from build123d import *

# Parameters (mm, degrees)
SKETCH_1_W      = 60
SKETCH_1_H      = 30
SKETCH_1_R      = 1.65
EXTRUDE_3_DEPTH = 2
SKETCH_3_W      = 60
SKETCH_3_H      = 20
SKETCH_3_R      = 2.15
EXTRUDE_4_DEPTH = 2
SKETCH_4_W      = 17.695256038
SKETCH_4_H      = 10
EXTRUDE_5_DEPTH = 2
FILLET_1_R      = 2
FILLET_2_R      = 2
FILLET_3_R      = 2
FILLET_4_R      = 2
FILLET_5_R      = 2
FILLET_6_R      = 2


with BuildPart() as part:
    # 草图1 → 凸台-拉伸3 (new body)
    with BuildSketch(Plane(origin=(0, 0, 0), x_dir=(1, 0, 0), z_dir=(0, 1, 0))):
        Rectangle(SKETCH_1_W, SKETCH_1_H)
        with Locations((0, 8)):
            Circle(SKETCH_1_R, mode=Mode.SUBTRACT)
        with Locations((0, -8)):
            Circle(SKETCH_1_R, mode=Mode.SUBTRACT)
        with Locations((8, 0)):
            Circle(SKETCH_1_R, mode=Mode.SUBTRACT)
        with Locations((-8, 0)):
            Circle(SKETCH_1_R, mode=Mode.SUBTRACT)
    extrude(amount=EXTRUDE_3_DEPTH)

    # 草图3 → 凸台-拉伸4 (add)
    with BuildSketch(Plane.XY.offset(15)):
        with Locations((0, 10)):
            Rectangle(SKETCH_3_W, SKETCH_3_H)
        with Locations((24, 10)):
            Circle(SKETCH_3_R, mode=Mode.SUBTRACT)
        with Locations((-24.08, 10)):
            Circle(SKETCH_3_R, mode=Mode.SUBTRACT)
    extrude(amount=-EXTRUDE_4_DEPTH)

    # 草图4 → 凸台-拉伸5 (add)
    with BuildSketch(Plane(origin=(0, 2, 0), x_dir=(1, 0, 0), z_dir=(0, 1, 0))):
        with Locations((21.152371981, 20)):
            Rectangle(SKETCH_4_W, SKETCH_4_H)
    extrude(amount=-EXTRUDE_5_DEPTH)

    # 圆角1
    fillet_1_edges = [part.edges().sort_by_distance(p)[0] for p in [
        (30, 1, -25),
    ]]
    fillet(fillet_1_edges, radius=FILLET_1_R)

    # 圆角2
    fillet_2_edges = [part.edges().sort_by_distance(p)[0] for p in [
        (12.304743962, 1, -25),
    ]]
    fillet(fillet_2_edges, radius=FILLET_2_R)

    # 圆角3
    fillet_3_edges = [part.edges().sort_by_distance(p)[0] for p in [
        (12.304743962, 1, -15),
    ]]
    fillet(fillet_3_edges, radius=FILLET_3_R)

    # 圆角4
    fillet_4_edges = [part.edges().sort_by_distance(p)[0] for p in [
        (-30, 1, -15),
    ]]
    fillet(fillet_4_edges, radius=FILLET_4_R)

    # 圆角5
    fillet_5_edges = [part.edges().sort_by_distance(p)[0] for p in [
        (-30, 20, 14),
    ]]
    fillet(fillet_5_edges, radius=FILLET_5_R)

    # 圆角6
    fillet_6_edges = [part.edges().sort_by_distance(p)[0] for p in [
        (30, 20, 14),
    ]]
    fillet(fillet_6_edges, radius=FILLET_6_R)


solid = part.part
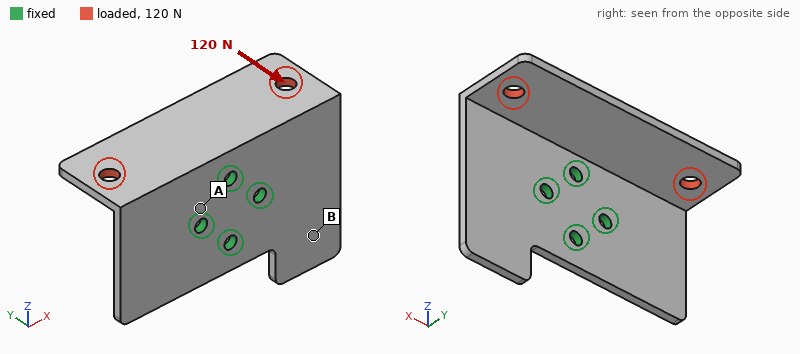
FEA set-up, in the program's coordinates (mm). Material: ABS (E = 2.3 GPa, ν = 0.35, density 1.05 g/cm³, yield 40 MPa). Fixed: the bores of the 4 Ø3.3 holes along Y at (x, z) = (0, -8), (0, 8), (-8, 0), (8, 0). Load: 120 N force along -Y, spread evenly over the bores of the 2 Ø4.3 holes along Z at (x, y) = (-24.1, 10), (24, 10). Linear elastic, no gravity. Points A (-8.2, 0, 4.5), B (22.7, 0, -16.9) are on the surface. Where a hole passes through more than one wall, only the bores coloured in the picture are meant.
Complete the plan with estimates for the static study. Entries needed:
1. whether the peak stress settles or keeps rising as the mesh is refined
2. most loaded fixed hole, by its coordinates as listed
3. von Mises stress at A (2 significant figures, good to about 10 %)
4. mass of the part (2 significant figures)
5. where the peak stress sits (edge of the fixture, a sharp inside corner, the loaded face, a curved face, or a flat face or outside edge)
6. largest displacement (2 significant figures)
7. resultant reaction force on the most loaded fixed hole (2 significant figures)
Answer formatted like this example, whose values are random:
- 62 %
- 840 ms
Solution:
- keeps rising
- (0, 8)
- 8.0 MPa
- 6.3 g
- edge of the fixture
- 0.82 mm
- 130 N
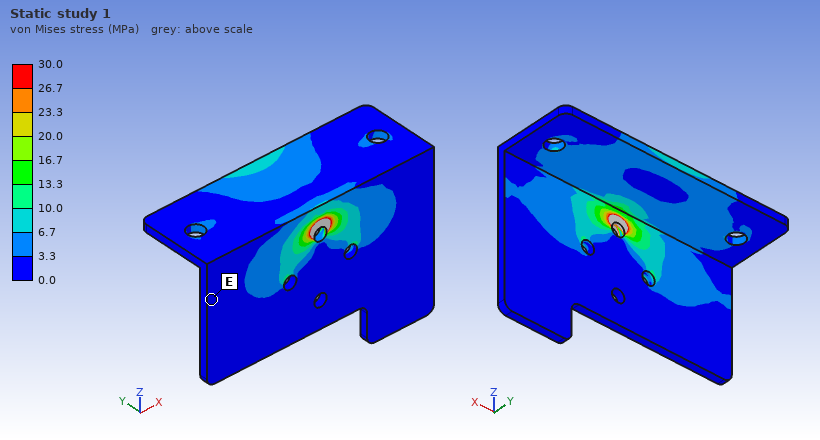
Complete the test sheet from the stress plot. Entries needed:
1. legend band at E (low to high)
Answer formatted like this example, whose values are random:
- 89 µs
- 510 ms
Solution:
- 0.0 to 3.3 MPa
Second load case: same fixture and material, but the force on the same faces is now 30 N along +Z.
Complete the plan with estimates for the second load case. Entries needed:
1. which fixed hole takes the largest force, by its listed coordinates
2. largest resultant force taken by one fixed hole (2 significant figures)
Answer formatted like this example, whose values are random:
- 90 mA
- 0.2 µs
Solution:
- (0, 8)
- 22 N
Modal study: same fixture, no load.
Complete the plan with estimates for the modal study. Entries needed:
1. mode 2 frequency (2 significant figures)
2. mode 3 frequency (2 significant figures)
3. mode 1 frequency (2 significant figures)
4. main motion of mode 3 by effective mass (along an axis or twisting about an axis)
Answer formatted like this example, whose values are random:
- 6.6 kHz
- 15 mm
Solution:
- 700 Hz
- 840 Hz
- 680 Hz
- along Z
